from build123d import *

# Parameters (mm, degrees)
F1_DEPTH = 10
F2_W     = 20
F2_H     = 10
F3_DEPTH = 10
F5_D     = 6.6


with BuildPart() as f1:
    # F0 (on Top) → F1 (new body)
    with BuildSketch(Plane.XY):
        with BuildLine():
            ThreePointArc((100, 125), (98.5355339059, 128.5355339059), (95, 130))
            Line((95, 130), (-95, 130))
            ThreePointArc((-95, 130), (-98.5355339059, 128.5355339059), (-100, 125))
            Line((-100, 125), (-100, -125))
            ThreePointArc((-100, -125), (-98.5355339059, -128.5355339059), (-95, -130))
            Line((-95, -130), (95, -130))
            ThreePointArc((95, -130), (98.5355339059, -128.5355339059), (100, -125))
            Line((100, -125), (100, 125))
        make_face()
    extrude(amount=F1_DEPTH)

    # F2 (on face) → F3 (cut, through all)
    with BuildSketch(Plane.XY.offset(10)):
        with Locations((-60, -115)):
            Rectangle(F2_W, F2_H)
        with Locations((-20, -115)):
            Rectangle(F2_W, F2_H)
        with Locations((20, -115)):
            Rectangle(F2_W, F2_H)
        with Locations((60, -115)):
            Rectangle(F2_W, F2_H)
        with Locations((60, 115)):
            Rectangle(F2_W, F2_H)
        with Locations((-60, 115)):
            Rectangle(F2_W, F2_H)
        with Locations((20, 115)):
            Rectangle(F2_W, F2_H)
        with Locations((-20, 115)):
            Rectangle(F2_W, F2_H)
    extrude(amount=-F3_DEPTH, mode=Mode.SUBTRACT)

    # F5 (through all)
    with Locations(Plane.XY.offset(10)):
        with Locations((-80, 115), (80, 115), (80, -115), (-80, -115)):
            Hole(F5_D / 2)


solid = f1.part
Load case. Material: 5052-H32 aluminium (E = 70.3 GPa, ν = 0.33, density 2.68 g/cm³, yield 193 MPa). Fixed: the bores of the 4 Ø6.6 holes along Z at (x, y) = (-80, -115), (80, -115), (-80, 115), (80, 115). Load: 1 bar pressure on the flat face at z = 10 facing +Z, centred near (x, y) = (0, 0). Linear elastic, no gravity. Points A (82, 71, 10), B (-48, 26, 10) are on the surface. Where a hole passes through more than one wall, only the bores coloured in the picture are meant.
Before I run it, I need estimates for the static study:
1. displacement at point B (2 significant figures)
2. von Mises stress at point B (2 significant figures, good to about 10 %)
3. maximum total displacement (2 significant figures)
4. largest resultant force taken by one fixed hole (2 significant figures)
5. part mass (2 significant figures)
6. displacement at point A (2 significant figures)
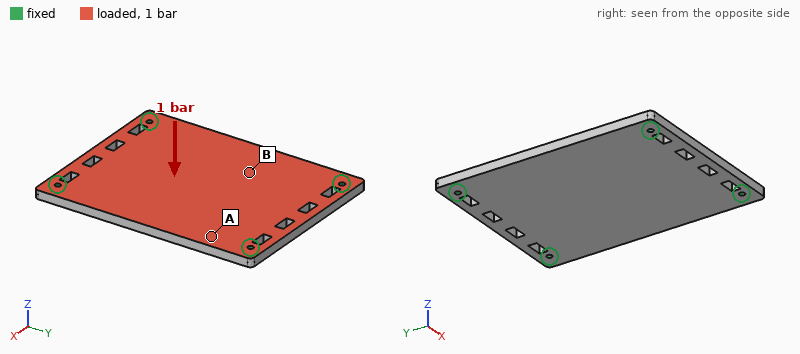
0.21 mm
15 MPa
0.24 mm
1.3 kN
1.3 kg
0.095 mm
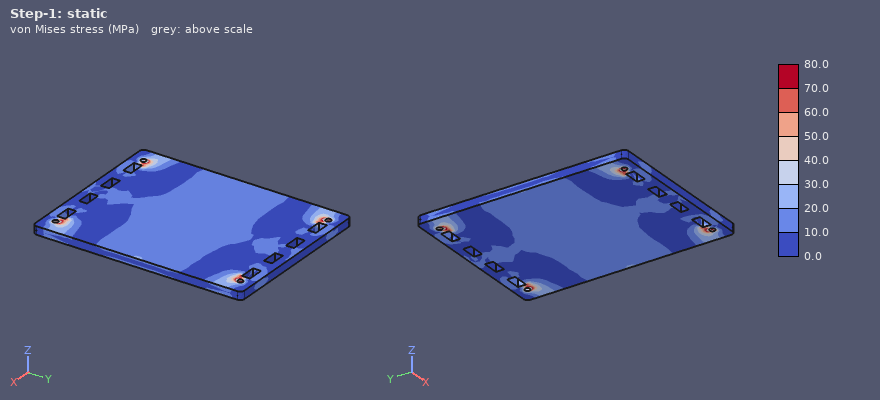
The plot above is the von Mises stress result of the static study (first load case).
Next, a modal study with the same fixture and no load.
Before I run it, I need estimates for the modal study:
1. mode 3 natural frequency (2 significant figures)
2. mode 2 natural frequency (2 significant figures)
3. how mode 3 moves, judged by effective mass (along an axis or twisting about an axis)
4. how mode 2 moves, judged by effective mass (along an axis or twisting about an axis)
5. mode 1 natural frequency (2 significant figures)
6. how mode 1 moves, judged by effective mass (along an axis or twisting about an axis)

1700 Hz
1100 Hz
twisting about X
twisting about Y
730 Hz
along Z
